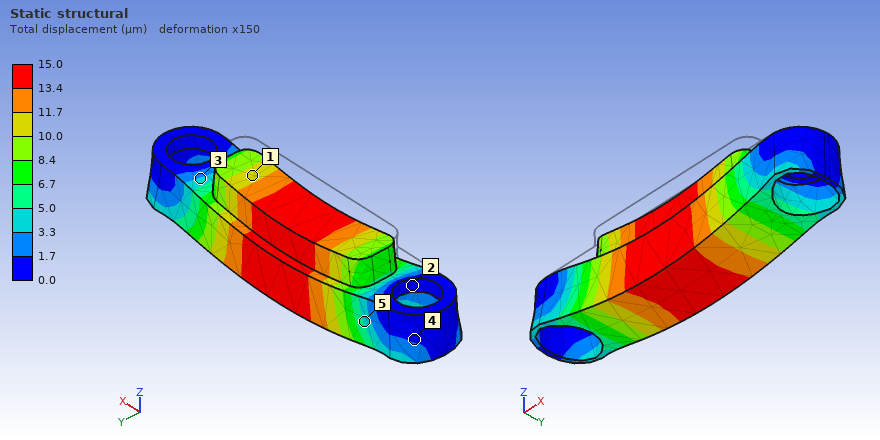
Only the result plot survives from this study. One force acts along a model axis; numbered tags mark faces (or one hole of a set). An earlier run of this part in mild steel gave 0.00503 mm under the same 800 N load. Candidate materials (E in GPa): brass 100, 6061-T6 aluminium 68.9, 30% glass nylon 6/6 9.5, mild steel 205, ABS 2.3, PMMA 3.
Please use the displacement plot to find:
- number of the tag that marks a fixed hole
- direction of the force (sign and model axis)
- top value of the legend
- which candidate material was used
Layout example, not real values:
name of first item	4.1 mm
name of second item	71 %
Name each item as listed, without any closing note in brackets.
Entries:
number of the tag that marks a fixed hole	2
direction of the force	-Z
top value of the legend	15.0 µm
which candidate material was used	6061-T6 aluminium
